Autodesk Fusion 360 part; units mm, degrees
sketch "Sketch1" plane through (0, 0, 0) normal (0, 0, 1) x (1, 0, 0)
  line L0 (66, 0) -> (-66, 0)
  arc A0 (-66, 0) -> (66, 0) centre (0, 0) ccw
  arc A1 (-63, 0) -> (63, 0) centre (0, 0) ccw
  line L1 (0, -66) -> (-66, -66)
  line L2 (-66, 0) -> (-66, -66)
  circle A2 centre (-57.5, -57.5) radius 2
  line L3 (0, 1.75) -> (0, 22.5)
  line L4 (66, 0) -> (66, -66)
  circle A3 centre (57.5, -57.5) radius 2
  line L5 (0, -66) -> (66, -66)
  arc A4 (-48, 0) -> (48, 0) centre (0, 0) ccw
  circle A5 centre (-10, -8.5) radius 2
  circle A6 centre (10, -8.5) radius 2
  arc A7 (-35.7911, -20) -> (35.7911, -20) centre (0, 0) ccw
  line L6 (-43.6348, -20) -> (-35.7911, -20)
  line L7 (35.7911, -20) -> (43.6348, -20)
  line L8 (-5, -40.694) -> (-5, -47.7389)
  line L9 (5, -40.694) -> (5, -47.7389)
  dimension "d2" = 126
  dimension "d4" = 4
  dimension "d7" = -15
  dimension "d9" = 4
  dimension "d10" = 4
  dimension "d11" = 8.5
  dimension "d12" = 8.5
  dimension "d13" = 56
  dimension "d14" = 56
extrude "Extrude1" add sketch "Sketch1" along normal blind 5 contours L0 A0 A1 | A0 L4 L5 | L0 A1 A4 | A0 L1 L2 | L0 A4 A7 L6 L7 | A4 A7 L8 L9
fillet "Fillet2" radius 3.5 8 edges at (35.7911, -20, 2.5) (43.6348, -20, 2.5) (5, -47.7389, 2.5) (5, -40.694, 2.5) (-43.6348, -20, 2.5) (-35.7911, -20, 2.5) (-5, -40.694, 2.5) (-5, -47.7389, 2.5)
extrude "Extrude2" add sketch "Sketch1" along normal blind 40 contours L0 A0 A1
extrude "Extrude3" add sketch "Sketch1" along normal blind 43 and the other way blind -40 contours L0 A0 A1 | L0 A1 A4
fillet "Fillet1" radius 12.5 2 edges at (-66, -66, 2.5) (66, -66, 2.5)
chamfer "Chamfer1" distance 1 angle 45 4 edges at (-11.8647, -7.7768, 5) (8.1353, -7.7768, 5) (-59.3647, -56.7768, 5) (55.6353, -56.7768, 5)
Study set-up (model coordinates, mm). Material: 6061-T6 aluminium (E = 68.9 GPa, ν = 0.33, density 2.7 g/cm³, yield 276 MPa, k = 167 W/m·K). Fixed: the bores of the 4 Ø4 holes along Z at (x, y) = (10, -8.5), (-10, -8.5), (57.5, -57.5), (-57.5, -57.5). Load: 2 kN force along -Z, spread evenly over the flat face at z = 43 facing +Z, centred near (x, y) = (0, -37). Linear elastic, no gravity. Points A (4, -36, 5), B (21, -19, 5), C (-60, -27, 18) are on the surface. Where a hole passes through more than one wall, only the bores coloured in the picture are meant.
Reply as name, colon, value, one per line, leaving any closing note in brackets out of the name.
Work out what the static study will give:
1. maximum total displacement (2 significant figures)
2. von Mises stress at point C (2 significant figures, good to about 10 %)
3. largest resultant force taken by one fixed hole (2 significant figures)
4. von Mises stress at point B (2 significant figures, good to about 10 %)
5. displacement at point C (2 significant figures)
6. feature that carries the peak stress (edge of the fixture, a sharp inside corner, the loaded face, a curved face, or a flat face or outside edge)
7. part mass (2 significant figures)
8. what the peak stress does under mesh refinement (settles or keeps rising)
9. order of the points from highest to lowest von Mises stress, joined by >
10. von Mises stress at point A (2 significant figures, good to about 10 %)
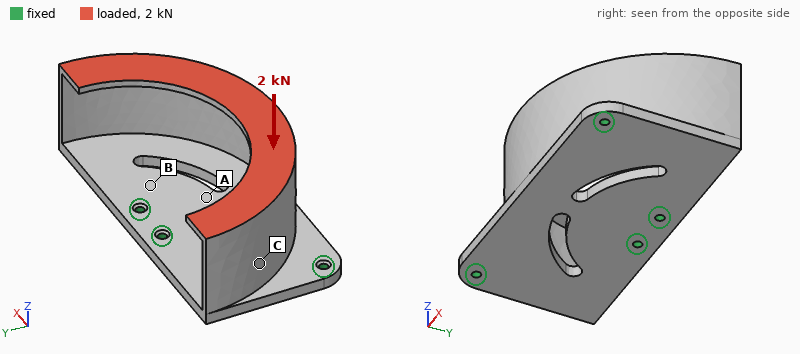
maximum total displacement: 0.34 mm
von Mises stress at point C: 7.1 MPa
largest resultant force taken by one fixed hole: 720 N
von Mises stress at point B: 26 MPa
displacement at point C: 0.13 mm
feature that carries the peak stress: edge of the fixture
part mass: 190 g
what the peak stress does under mesh refinement: keeps rising
order of the points from highest to lowest von Mises stress, joined by >: B > A > C
von Mises stress at point A: 12 MPa
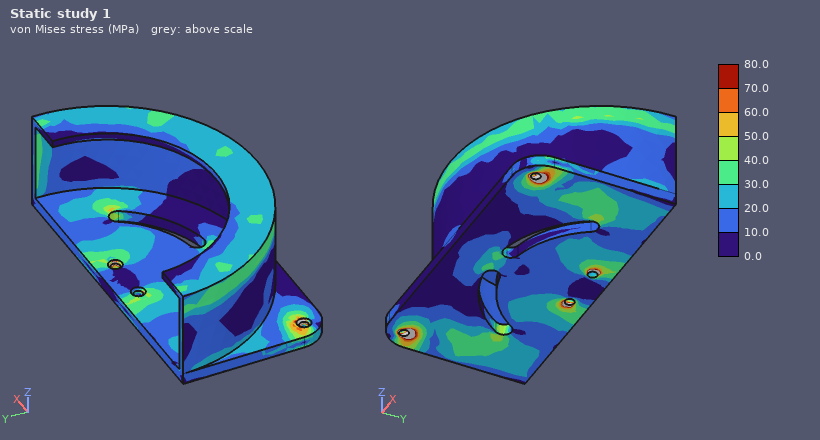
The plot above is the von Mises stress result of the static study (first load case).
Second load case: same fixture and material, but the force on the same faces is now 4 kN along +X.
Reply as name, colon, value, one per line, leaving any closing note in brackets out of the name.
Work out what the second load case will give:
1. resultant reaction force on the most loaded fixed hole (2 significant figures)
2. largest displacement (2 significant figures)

resultant reaction force on the most loaded fixed hole: 2.2 kN
largest displacement: 1.1 mm
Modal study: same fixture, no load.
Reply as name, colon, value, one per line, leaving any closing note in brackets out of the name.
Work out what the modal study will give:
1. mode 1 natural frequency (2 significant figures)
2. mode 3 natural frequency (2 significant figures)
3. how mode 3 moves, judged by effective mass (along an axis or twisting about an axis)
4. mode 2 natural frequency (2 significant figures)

mode 1 natural frequency: 1100 Hz
mode 3 natural frequency: 2400 Hz
how mode 3 moves, judged by effective mass: along Z
mode 2 natural frequency: 1400 Hz
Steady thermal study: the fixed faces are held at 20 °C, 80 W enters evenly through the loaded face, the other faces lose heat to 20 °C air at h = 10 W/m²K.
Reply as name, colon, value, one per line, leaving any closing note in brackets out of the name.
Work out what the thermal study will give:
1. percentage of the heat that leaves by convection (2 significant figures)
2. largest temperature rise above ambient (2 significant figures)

percentage of the heat that leaves by convection: 12 %
largest temperature rise above ambient: 55 K
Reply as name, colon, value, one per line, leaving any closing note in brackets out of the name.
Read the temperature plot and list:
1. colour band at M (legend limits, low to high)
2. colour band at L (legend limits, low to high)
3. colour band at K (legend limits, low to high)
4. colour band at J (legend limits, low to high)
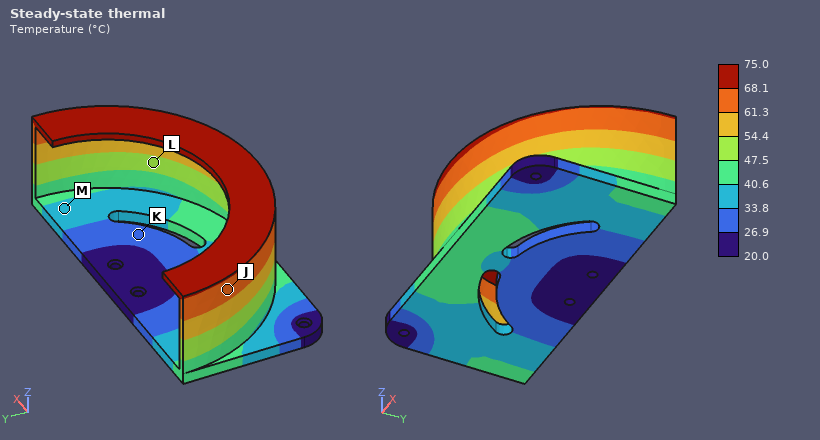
colour band at M: 33.8 to 40.6 °C
colour band at L: 47.5 to 54.4 °C
colour band at K: 26.9 to 33.8 °C
colour band at J: 61.3 to 68.1 °C
